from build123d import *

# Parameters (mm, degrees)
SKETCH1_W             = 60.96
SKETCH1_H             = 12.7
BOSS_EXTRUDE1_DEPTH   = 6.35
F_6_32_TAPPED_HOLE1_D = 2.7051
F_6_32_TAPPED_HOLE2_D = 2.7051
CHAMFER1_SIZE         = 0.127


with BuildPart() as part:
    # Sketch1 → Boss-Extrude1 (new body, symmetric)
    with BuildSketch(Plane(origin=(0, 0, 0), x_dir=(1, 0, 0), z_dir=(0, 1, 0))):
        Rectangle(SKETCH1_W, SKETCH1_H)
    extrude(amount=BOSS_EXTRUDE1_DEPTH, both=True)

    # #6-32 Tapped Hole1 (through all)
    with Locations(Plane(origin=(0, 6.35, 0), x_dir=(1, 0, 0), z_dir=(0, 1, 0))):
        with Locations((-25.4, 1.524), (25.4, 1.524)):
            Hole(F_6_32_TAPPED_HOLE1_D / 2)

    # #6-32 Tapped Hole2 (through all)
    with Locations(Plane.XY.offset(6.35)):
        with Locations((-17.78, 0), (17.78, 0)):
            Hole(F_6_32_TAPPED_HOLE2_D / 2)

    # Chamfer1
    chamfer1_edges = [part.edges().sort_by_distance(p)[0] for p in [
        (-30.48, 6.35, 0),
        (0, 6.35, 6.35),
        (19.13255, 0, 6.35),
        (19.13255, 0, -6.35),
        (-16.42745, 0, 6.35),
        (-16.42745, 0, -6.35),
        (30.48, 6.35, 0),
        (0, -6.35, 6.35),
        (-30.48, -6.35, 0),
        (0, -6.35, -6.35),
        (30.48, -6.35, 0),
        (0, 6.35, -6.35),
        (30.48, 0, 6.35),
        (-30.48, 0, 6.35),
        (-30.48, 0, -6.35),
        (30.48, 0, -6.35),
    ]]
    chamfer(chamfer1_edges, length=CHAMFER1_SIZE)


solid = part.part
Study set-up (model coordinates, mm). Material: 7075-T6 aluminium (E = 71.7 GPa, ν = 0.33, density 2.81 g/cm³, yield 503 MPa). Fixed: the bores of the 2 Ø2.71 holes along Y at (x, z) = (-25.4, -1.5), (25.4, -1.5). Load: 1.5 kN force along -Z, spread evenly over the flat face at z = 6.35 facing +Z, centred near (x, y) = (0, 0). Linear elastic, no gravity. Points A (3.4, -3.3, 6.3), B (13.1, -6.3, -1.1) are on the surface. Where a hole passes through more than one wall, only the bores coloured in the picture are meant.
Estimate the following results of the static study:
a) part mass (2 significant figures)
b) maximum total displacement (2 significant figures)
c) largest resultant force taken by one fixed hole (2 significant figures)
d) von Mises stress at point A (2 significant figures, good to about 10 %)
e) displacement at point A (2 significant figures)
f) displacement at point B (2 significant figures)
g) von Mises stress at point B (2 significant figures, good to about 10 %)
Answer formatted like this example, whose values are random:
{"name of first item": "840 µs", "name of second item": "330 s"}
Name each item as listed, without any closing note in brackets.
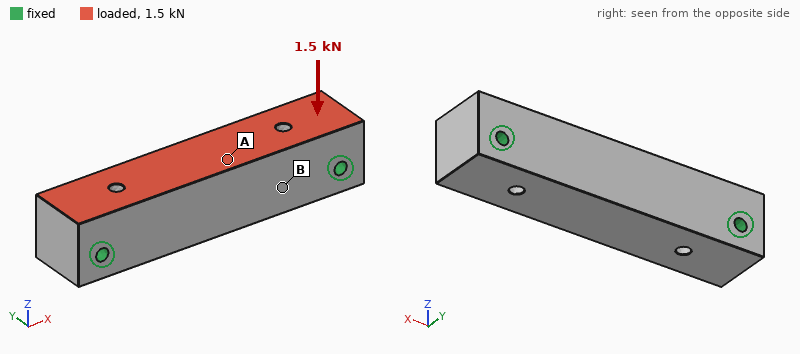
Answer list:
{"part mass": "27 g", "maximum total displacement": "8.7 µm", "largest resultant force taken by one fixed hole": "790 N", "von Mises stress at point A": "14 MPa", "displacement at point A": "8.3 µm", "displacement at point B": "5.8 µm", "von Mises stress at point B": "6.0 MPa"}
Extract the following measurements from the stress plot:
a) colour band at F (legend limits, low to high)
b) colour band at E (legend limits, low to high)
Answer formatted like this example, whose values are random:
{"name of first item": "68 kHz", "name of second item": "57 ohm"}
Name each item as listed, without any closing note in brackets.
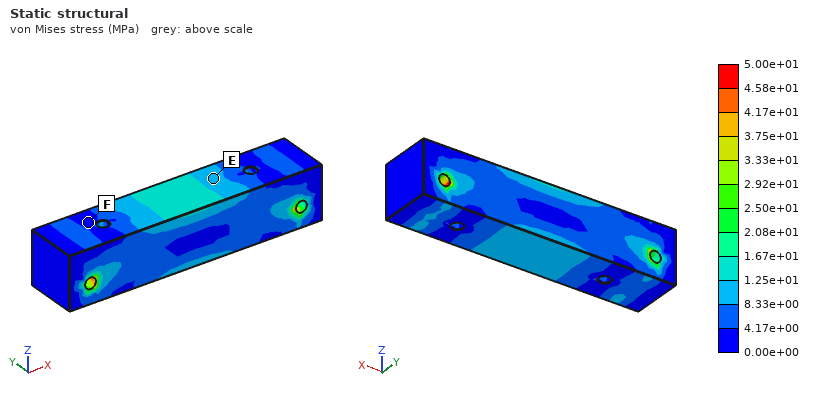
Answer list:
{"colour band at F": "0.00e+00 to 4.17e+00 MPa", "colour band at E": "8.33e+00 to 1.25e+01 MPa"}
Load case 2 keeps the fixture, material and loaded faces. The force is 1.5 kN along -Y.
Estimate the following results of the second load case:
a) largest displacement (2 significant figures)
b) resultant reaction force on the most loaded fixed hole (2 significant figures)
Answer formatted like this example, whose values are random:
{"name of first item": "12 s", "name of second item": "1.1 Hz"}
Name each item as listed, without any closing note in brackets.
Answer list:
{"largest displacement": "12 µm", "resultant reaction force on the most loaded fixed hole": "750 N"}
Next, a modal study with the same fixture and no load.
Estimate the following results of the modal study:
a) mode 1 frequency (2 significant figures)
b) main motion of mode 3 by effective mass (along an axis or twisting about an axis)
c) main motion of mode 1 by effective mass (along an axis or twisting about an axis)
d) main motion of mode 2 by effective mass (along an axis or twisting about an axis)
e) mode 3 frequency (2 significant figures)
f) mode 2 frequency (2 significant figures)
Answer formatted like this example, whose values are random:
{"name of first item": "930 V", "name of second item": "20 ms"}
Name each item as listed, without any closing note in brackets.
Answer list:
{"mode 1 frequency": "14 kHz", "main motion of mode 3 by effective mass": "twisting about X", "main motion of mode 1 by effective mass": "along Z", "main motion of mode 2 by effective mass": "along Y", "mode 3 frequency": "26 kHz", "mode 2 frequency": "17 kHz"}
